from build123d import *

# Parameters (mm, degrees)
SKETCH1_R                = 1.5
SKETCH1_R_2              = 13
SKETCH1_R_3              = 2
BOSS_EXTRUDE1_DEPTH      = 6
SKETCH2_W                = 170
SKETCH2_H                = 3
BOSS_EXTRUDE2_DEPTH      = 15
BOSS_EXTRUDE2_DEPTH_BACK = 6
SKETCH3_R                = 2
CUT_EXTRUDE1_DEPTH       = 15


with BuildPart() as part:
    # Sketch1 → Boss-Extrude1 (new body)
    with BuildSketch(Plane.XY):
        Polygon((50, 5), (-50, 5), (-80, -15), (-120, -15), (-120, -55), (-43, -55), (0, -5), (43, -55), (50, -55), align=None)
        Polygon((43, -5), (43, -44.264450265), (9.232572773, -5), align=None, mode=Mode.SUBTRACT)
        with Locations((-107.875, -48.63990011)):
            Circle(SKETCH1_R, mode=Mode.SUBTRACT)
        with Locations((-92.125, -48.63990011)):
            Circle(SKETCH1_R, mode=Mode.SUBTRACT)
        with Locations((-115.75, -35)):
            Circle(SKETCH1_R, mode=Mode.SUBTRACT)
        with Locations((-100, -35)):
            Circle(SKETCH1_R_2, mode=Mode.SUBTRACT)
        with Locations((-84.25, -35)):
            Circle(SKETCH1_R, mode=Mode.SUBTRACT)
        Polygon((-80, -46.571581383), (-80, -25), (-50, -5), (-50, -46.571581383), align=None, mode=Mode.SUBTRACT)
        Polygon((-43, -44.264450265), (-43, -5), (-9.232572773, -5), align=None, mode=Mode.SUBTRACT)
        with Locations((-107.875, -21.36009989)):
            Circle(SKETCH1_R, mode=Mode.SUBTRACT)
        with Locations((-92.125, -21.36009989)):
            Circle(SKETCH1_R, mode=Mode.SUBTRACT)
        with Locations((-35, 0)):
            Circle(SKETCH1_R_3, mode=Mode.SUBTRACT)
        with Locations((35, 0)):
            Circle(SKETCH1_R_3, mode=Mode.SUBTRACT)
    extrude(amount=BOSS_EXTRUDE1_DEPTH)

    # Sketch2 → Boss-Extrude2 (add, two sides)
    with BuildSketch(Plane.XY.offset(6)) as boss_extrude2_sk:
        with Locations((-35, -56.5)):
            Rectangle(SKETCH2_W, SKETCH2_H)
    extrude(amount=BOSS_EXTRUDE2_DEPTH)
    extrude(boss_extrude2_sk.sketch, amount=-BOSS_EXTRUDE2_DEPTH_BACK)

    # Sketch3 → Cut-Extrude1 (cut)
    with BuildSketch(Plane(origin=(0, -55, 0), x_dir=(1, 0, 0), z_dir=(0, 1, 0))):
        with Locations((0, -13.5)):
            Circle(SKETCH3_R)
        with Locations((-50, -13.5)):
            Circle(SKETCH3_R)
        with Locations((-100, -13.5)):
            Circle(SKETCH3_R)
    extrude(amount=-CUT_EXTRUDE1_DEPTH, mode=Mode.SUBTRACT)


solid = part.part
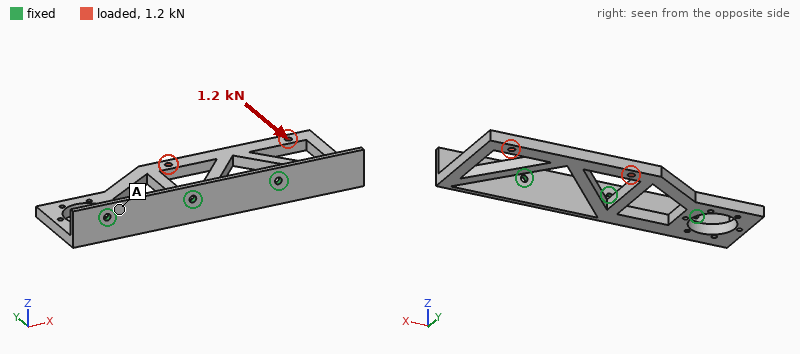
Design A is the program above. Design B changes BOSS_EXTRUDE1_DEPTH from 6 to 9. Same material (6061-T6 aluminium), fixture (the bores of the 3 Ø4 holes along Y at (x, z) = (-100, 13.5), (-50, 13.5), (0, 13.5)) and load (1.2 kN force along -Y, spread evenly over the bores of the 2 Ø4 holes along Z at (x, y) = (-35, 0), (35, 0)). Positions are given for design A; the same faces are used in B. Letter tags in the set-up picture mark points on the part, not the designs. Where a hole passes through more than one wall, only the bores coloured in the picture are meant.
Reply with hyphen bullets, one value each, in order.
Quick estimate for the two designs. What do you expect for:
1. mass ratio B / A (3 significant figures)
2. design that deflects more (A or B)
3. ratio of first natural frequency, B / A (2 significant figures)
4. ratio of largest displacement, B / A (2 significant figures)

- 1.35
- A
- 1.1
- 0.62
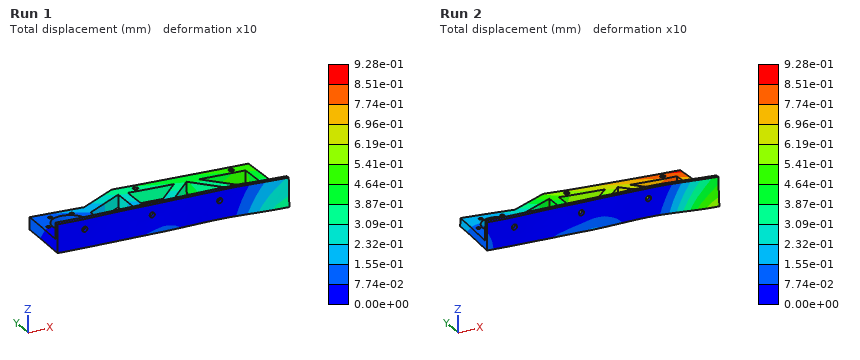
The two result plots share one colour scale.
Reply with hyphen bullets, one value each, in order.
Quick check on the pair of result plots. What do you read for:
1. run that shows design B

- Run 1
